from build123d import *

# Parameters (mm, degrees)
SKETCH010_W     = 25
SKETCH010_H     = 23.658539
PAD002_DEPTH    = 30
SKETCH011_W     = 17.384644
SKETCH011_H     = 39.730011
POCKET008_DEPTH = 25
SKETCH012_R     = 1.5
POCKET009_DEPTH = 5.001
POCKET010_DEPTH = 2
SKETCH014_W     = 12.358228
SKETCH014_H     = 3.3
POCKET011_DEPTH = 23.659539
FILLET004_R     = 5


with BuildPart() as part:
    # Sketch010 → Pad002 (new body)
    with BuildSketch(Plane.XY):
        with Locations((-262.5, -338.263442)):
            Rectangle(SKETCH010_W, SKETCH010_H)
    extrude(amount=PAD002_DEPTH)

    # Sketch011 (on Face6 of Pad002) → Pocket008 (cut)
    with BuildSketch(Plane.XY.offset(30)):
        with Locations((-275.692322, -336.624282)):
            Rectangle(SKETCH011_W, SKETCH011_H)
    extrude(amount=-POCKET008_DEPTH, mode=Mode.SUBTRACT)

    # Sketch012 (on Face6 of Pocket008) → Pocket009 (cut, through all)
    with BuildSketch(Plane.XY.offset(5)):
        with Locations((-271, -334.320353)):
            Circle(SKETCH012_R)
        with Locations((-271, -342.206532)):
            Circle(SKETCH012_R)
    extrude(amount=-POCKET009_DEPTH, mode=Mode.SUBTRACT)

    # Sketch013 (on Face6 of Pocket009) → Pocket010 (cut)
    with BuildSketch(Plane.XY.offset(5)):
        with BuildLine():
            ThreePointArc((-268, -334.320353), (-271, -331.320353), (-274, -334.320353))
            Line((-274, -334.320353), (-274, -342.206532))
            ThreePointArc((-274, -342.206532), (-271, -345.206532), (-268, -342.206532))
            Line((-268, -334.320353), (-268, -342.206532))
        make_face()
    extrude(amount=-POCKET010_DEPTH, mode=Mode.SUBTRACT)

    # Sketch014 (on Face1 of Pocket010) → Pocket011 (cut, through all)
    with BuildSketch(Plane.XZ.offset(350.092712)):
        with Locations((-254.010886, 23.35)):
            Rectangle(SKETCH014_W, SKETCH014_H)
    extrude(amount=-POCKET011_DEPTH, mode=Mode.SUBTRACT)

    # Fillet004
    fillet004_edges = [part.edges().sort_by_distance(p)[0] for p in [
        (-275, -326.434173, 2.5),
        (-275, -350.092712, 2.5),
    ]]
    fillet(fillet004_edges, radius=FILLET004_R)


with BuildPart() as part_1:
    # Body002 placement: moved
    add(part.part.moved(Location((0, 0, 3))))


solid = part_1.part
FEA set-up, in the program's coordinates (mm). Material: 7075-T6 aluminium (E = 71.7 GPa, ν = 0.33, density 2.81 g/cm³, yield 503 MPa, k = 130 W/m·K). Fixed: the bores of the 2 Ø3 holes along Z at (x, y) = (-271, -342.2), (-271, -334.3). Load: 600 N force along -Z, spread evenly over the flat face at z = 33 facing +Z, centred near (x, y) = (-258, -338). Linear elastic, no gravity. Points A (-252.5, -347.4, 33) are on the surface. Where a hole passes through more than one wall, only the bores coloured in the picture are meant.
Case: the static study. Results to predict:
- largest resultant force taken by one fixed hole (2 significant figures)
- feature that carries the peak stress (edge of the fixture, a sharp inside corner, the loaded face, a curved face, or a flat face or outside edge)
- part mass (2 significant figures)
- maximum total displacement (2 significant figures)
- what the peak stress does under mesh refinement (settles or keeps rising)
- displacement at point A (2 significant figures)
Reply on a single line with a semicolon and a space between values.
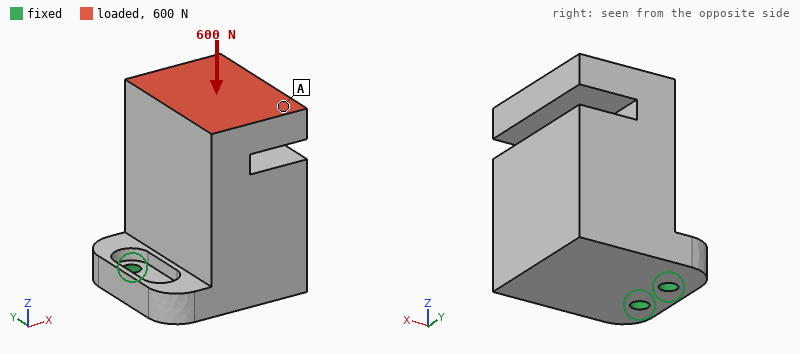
300 N; edge of the fixture; 34 g; 0.19 mm; keeps rising; 0.18 mm
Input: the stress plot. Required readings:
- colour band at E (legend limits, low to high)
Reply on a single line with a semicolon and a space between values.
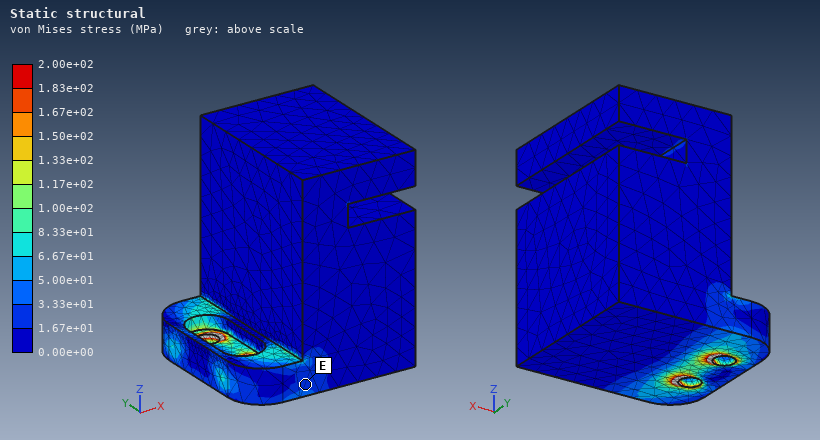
1.67e+01 to 3.33e+01 MPa
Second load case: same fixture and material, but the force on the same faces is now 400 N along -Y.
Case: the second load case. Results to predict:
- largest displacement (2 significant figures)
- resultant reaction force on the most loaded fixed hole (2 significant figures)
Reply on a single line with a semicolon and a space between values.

72 µm; 1.1 kN
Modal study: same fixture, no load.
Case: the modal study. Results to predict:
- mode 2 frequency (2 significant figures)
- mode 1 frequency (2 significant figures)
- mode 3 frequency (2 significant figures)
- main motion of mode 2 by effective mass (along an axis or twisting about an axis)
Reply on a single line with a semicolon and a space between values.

3700 Hz; 1600 Hz; 8500 Hz; along Y
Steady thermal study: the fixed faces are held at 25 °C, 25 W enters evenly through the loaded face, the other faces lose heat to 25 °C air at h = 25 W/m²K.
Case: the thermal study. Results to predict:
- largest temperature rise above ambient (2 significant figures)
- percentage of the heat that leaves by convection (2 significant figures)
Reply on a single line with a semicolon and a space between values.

40 K; 7.5 %
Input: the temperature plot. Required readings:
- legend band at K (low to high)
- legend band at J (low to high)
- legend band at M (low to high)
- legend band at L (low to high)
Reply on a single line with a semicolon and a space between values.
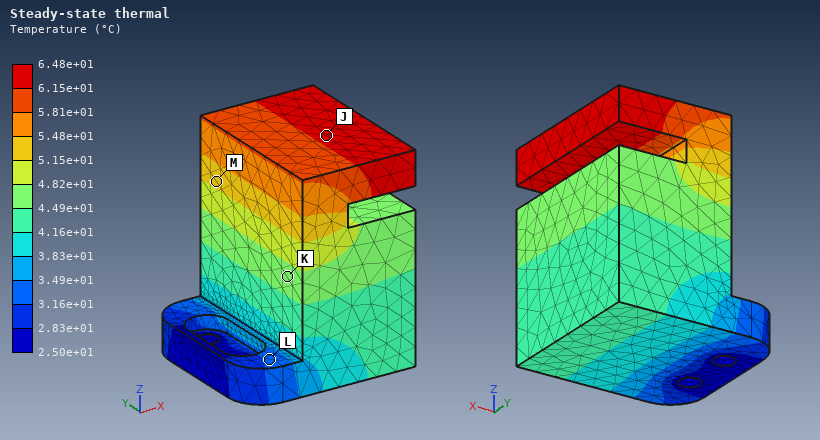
4.49e+01 to 4.82e+01 °C; 6.15e+01 to 6.48e+01 °C; 5.15e+01 to 5.48e+01 °C; 3.16e+01 to 3.49e+01 °C
